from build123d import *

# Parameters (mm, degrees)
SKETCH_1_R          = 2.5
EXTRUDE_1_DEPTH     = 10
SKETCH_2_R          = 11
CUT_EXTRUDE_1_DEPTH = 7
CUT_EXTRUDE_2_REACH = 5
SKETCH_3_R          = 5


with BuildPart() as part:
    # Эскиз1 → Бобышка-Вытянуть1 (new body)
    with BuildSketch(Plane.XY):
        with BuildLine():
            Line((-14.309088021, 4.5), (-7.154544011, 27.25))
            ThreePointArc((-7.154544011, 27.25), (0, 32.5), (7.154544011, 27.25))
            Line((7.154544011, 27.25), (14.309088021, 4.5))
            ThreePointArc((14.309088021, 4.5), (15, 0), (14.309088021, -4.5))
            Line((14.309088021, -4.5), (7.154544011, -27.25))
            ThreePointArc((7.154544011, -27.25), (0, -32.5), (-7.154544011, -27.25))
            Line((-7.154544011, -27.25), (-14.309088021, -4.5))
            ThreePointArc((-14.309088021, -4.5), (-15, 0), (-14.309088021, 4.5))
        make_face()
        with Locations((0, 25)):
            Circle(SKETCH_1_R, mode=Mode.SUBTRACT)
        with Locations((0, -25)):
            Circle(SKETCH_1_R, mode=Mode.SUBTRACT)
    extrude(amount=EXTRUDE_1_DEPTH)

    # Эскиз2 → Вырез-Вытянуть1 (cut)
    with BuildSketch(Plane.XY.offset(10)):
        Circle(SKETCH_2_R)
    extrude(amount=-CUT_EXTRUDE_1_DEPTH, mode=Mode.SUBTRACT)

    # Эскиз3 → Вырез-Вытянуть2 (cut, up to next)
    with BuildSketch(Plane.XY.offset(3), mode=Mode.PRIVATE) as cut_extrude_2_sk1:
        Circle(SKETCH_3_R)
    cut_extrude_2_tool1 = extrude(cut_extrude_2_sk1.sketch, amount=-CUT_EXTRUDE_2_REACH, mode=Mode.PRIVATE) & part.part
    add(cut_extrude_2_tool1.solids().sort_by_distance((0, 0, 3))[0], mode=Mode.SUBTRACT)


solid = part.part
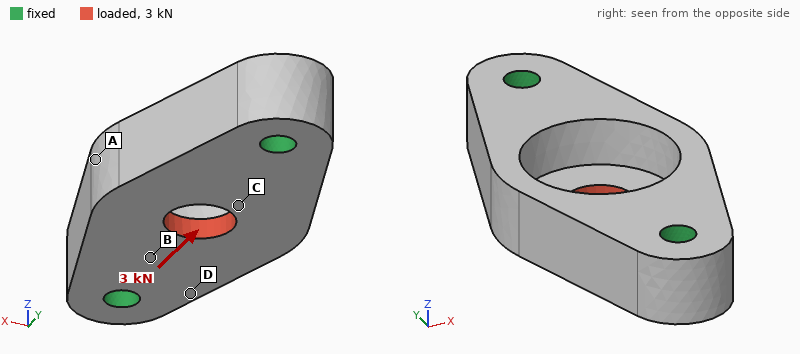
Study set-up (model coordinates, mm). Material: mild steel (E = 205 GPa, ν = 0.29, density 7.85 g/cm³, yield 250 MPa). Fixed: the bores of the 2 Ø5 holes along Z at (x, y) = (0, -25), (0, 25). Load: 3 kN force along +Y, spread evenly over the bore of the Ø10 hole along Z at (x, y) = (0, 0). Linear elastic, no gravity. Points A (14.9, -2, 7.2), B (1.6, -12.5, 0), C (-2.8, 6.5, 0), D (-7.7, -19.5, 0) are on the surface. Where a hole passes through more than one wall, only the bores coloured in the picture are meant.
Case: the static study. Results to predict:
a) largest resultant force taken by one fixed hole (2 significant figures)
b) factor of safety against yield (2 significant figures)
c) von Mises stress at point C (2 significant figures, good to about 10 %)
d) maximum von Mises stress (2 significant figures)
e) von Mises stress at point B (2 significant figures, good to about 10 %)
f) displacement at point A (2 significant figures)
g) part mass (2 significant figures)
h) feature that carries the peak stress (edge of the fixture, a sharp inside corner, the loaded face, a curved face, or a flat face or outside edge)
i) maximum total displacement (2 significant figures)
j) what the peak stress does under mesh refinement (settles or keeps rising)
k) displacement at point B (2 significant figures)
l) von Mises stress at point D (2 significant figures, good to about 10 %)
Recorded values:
1.5 kN
4.4
33 MPa
57 MPa
27 MPa
0.66 µm
80 g
the loaded face
2.4 µm
settles
1.1 µm
9.6 MPa
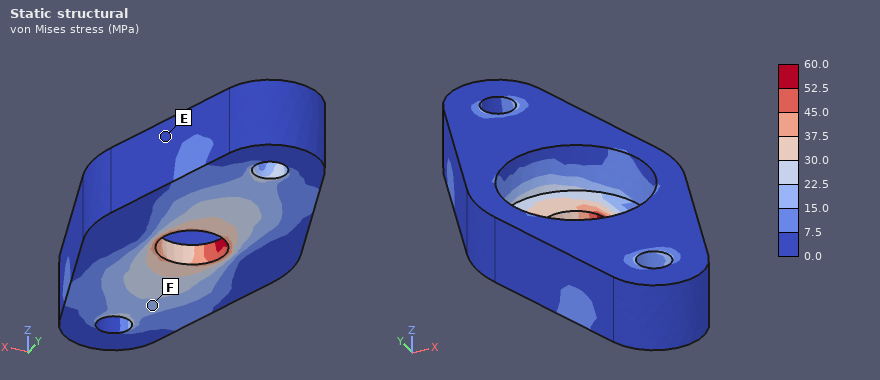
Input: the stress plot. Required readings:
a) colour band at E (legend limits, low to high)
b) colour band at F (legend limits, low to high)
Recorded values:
0.0 to 7.5 MPa
15.0 to 22.5 MPa
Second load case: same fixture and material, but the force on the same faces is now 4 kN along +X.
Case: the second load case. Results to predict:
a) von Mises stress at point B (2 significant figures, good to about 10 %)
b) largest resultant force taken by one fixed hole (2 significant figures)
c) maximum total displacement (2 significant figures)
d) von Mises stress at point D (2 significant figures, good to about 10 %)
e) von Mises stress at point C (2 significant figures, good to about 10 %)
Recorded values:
31 MPa
2.0 kN
9.5 µm
26 MPa
41 MPa
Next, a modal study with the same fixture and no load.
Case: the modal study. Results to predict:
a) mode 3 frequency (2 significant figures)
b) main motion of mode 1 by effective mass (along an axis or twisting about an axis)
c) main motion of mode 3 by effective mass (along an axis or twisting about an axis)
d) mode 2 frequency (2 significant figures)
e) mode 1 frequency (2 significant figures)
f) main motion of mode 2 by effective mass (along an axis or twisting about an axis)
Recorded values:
25 kHz
along Z
along X
17 kHz
16 kHz
twisting about Y
